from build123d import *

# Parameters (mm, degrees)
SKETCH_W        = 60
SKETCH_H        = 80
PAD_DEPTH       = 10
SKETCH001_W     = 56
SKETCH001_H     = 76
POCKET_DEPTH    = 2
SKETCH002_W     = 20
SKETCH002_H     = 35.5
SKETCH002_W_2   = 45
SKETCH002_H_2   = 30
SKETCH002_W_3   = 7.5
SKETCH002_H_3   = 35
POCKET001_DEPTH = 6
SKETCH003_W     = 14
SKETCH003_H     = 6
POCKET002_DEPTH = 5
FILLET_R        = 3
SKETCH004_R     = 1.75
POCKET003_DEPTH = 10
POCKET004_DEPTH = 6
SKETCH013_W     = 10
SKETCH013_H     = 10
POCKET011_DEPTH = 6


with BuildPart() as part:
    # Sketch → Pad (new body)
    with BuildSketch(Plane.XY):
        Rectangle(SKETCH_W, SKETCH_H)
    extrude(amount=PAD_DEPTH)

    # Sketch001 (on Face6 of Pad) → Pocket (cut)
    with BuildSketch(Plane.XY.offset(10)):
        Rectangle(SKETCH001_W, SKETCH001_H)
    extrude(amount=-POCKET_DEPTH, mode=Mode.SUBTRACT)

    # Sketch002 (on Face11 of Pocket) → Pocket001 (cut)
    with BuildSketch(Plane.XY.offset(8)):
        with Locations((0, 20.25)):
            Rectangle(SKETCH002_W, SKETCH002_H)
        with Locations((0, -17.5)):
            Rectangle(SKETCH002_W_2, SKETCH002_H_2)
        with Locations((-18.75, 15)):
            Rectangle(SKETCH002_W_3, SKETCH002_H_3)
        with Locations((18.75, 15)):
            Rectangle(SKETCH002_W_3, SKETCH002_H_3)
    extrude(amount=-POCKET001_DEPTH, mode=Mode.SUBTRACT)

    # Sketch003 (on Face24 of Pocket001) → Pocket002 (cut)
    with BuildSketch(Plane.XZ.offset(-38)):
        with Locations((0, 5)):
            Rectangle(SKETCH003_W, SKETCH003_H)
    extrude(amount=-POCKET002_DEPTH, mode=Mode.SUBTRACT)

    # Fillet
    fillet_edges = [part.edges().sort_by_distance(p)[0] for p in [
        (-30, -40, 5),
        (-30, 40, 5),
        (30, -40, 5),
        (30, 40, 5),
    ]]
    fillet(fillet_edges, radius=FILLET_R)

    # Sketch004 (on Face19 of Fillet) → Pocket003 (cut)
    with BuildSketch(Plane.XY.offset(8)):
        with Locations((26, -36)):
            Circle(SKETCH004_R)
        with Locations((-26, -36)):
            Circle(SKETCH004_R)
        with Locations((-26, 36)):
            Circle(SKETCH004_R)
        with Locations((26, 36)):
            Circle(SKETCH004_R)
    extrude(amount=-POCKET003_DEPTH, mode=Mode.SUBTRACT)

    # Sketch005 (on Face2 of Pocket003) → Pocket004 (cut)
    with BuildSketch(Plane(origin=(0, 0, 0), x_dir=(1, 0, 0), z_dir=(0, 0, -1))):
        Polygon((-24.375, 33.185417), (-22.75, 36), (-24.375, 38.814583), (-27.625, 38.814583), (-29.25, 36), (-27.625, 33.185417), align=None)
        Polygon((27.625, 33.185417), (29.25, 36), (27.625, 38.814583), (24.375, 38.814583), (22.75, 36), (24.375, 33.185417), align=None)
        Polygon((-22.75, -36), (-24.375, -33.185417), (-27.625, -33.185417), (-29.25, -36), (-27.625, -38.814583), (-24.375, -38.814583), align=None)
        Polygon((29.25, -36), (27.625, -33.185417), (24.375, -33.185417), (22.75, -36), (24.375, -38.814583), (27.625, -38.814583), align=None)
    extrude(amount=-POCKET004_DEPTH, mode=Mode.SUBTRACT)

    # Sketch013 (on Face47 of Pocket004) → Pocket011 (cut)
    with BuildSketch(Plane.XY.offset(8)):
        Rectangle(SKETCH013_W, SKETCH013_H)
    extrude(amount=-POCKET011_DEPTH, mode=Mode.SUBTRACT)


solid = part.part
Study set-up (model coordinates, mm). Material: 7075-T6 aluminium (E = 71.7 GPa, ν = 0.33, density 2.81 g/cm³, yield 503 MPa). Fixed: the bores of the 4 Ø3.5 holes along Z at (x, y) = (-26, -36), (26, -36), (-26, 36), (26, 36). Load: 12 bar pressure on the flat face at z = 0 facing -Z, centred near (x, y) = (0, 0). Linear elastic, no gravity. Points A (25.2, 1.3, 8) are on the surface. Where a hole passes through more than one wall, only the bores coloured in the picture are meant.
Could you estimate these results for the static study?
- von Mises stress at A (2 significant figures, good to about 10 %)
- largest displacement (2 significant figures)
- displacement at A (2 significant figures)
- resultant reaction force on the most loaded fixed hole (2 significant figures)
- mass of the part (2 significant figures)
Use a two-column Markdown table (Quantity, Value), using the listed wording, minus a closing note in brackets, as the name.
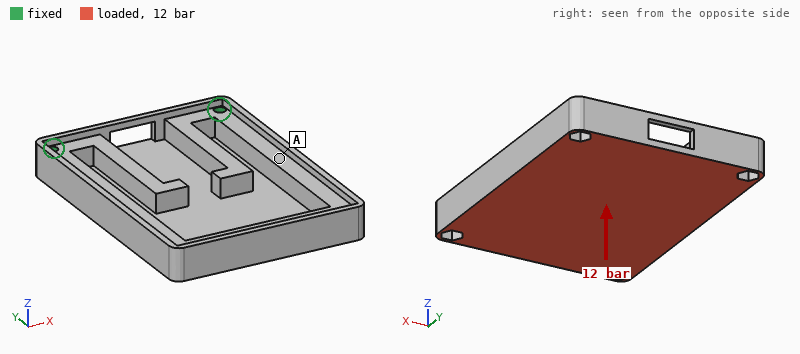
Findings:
| Quantity | Value |
|---|---|
| von Mises stress at A | 53 MPa |
| largest displacement | 0.32 mm |
| displacement at A | 0.11 mm |
| resultant reaction force on the most loaded fixed hole | 3.0 kN |
| mass of the part | 64 g |
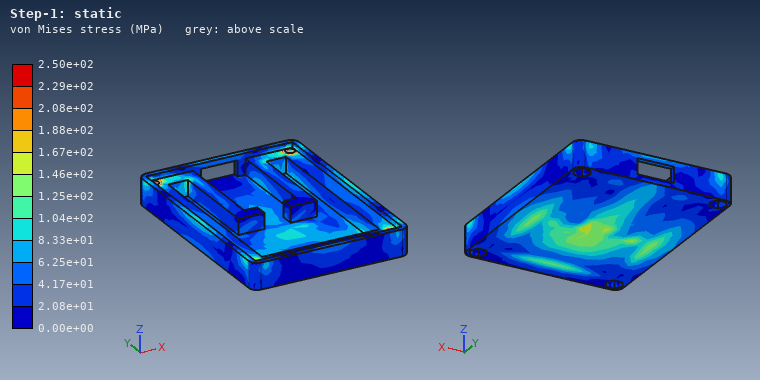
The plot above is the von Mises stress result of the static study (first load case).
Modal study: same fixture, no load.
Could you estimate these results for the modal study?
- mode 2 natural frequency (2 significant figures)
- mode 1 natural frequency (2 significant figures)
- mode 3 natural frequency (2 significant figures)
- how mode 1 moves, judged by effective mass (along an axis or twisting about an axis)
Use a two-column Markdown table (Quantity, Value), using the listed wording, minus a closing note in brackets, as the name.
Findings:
| Quantity | Value |
|---|---|
| mode 2 natural frequency | 5600 Hz |
| mode 1 natural frequency | 4300 Hz |
| mode 3 natural frequency | 7200 Hz |
| how mode 1 moves, judged by effective mass | along Z |
